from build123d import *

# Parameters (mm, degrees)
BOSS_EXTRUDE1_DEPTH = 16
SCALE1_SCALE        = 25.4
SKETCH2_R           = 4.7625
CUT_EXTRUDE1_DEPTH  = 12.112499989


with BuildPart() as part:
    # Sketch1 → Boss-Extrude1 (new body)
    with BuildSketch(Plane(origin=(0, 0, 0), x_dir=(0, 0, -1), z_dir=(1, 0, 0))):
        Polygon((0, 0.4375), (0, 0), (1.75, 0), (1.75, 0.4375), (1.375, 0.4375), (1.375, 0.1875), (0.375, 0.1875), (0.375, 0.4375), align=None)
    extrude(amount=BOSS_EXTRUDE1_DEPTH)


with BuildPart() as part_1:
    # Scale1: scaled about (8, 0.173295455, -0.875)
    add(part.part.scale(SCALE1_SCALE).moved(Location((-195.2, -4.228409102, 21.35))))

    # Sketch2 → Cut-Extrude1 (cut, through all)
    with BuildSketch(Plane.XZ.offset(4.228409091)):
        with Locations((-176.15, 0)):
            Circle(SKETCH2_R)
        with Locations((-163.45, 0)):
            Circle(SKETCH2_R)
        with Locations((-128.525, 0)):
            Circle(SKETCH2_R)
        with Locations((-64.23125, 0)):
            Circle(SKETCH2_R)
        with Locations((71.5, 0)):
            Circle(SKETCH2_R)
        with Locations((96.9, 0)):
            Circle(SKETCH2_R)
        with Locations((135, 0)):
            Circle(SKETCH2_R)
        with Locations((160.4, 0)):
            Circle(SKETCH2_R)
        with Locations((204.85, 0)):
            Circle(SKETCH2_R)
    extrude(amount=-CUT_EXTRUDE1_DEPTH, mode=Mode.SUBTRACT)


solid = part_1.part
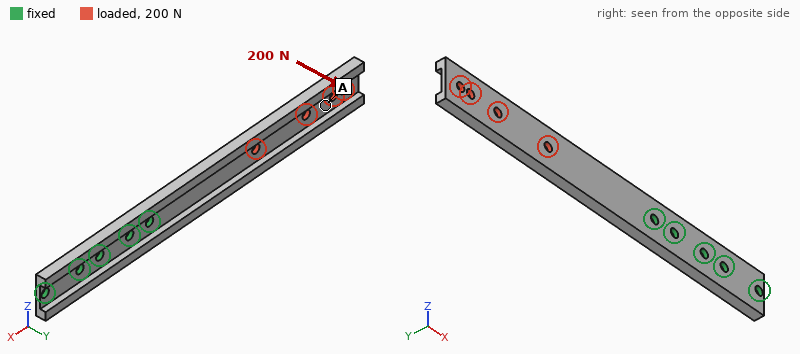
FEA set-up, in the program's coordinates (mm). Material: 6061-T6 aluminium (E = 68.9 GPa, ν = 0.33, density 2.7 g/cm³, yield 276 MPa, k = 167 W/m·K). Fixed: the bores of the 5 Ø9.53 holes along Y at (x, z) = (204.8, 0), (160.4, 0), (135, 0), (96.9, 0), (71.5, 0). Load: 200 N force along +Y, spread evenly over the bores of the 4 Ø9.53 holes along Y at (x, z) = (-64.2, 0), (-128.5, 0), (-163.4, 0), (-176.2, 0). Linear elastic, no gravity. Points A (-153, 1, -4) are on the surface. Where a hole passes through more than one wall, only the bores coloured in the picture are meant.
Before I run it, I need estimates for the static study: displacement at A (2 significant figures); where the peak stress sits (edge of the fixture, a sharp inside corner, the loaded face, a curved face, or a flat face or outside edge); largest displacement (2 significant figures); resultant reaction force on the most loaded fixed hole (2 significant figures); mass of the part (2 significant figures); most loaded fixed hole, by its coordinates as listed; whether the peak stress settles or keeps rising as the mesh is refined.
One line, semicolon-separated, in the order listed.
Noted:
3.3 mm; edge of the fixture; 4.2 mm; 1.9 kN; 360 g; (71.5, 0); keeps rising
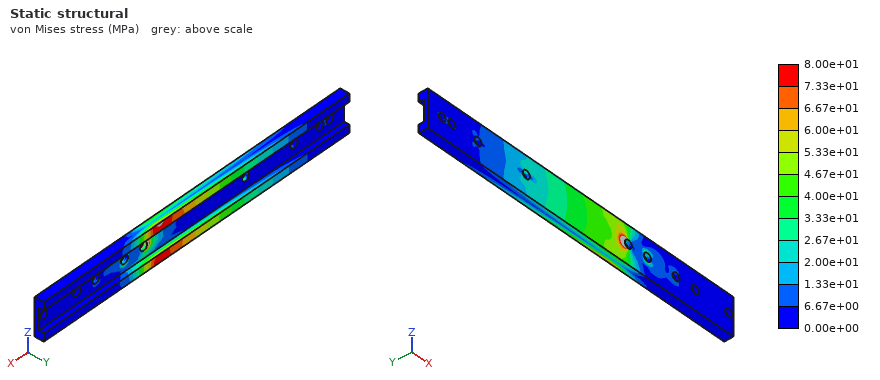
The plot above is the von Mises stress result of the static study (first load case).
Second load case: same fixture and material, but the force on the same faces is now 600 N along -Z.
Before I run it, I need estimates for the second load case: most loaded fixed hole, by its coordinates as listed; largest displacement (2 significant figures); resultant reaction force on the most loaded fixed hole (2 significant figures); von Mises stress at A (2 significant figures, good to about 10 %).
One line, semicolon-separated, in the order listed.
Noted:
(71.5, 0); 0.73 mm; 2.7 kN; 5.1 MPa
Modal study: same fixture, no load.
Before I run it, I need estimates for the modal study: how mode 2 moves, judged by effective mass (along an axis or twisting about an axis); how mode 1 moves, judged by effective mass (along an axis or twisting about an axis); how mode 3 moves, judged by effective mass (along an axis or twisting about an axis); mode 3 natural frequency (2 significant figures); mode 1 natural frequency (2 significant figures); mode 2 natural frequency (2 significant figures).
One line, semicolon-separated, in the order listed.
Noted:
along Z; along Y; twisting about X; 710 Hz; 120 Hz; 480 Hz
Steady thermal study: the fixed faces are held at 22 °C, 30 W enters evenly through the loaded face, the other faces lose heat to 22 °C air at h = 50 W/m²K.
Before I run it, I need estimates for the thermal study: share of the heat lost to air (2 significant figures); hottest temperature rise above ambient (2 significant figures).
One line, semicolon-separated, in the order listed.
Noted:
85 %; 33 K
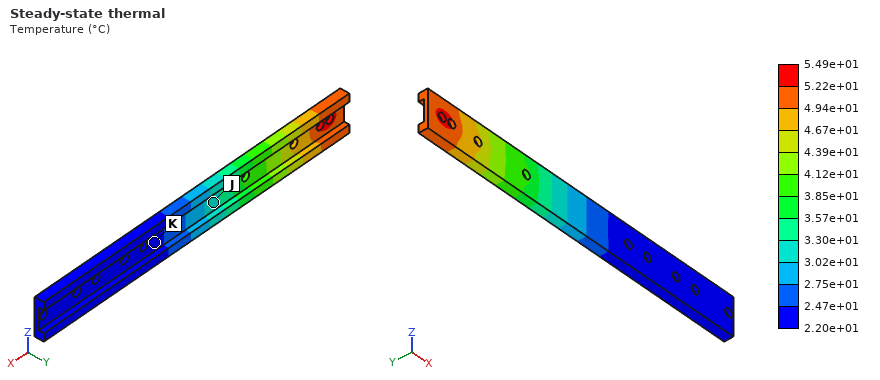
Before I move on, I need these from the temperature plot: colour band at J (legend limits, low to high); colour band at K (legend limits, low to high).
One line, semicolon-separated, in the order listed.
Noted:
3.02e+01 to 3.30e+01 °C; 2.20e+01 to 2.47e+01 °C
